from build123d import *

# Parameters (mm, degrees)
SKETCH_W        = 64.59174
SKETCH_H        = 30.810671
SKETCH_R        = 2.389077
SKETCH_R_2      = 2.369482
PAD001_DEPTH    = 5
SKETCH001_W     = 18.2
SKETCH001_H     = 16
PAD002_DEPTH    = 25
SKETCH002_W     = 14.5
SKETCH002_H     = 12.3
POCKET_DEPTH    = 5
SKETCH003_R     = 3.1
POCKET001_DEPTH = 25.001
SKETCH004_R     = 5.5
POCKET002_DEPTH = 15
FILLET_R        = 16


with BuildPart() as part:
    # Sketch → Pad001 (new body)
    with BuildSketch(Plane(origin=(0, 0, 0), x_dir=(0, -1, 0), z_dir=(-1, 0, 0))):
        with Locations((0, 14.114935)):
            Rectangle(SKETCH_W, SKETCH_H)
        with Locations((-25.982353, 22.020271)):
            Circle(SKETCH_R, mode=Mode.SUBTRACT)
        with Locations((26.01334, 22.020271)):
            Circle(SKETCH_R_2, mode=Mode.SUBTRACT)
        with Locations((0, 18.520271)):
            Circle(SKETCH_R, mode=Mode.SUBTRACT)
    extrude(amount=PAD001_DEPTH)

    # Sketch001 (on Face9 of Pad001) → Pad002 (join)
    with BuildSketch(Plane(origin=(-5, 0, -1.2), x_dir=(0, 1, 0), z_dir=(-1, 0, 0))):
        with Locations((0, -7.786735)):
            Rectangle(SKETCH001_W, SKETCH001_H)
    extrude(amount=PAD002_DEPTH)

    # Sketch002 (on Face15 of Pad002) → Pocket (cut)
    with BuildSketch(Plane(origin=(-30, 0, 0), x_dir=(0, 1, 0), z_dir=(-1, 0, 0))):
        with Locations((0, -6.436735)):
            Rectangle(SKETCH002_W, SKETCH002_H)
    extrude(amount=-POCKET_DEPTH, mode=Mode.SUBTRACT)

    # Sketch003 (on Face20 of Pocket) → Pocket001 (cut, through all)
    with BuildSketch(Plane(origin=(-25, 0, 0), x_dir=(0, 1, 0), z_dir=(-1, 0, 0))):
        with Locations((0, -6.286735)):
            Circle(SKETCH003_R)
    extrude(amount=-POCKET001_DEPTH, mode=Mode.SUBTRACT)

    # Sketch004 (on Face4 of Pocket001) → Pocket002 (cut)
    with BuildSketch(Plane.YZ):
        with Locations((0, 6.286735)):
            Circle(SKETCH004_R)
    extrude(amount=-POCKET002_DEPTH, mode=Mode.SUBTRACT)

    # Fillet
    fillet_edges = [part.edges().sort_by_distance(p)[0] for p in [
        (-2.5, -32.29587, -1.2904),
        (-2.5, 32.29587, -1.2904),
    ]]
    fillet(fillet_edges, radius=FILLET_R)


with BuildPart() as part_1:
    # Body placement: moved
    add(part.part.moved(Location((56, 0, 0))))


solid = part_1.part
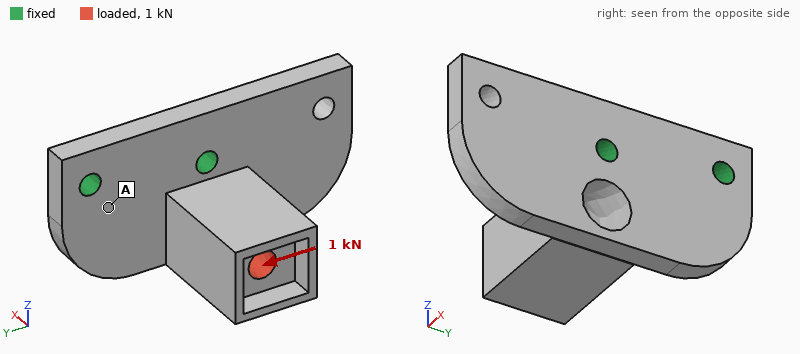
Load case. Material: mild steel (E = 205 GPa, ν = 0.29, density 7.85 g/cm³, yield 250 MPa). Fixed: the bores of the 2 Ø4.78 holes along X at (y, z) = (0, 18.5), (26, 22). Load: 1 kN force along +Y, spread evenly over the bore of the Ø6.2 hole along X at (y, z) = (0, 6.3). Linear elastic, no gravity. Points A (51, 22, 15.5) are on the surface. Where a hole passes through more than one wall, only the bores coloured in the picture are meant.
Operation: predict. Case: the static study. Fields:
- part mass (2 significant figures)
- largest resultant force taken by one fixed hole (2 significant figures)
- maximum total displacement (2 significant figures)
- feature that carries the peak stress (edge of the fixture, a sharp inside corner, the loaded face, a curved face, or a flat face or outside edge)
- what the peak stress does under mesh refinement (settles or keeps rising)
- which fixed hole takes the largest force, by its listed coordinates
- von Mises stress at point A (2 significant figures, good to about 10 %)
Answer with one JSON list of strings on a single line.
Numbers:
["110 g", "890 N", "27 µm", "edge of the fixture", "keeps rising", "(0, 18.5)", "11 MPa"]
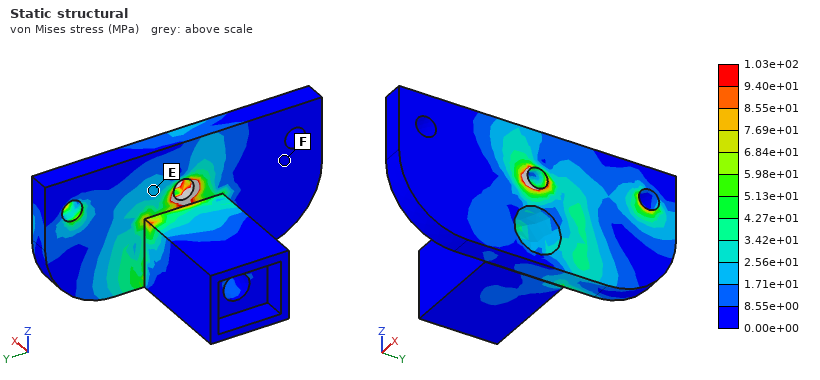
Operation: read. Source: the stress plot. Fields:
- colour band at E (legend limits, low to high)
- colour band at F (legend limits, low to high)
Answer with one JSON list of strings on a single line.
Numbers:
["1.71e+01 to 2.56e+01 MPa", "0.00e+00 to 8.55e+00 MPa"]
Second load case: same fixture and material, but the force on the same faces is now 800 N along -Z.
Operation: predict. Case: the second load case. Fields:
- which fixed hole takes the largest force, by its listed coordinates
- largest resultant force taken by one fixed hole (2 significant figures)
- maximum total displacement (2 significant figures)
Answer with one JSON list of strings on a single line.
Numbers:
["(0, 18.5)", "780 N", "54 µm"]
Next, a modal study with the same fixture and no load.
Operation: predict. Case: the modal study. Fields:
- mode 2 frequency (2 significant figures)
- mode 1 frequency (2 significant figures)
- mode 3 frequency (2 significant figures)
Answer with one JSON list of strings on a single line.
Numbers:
["4300 Hz", "3600 Hz", "7400 Hz"]
